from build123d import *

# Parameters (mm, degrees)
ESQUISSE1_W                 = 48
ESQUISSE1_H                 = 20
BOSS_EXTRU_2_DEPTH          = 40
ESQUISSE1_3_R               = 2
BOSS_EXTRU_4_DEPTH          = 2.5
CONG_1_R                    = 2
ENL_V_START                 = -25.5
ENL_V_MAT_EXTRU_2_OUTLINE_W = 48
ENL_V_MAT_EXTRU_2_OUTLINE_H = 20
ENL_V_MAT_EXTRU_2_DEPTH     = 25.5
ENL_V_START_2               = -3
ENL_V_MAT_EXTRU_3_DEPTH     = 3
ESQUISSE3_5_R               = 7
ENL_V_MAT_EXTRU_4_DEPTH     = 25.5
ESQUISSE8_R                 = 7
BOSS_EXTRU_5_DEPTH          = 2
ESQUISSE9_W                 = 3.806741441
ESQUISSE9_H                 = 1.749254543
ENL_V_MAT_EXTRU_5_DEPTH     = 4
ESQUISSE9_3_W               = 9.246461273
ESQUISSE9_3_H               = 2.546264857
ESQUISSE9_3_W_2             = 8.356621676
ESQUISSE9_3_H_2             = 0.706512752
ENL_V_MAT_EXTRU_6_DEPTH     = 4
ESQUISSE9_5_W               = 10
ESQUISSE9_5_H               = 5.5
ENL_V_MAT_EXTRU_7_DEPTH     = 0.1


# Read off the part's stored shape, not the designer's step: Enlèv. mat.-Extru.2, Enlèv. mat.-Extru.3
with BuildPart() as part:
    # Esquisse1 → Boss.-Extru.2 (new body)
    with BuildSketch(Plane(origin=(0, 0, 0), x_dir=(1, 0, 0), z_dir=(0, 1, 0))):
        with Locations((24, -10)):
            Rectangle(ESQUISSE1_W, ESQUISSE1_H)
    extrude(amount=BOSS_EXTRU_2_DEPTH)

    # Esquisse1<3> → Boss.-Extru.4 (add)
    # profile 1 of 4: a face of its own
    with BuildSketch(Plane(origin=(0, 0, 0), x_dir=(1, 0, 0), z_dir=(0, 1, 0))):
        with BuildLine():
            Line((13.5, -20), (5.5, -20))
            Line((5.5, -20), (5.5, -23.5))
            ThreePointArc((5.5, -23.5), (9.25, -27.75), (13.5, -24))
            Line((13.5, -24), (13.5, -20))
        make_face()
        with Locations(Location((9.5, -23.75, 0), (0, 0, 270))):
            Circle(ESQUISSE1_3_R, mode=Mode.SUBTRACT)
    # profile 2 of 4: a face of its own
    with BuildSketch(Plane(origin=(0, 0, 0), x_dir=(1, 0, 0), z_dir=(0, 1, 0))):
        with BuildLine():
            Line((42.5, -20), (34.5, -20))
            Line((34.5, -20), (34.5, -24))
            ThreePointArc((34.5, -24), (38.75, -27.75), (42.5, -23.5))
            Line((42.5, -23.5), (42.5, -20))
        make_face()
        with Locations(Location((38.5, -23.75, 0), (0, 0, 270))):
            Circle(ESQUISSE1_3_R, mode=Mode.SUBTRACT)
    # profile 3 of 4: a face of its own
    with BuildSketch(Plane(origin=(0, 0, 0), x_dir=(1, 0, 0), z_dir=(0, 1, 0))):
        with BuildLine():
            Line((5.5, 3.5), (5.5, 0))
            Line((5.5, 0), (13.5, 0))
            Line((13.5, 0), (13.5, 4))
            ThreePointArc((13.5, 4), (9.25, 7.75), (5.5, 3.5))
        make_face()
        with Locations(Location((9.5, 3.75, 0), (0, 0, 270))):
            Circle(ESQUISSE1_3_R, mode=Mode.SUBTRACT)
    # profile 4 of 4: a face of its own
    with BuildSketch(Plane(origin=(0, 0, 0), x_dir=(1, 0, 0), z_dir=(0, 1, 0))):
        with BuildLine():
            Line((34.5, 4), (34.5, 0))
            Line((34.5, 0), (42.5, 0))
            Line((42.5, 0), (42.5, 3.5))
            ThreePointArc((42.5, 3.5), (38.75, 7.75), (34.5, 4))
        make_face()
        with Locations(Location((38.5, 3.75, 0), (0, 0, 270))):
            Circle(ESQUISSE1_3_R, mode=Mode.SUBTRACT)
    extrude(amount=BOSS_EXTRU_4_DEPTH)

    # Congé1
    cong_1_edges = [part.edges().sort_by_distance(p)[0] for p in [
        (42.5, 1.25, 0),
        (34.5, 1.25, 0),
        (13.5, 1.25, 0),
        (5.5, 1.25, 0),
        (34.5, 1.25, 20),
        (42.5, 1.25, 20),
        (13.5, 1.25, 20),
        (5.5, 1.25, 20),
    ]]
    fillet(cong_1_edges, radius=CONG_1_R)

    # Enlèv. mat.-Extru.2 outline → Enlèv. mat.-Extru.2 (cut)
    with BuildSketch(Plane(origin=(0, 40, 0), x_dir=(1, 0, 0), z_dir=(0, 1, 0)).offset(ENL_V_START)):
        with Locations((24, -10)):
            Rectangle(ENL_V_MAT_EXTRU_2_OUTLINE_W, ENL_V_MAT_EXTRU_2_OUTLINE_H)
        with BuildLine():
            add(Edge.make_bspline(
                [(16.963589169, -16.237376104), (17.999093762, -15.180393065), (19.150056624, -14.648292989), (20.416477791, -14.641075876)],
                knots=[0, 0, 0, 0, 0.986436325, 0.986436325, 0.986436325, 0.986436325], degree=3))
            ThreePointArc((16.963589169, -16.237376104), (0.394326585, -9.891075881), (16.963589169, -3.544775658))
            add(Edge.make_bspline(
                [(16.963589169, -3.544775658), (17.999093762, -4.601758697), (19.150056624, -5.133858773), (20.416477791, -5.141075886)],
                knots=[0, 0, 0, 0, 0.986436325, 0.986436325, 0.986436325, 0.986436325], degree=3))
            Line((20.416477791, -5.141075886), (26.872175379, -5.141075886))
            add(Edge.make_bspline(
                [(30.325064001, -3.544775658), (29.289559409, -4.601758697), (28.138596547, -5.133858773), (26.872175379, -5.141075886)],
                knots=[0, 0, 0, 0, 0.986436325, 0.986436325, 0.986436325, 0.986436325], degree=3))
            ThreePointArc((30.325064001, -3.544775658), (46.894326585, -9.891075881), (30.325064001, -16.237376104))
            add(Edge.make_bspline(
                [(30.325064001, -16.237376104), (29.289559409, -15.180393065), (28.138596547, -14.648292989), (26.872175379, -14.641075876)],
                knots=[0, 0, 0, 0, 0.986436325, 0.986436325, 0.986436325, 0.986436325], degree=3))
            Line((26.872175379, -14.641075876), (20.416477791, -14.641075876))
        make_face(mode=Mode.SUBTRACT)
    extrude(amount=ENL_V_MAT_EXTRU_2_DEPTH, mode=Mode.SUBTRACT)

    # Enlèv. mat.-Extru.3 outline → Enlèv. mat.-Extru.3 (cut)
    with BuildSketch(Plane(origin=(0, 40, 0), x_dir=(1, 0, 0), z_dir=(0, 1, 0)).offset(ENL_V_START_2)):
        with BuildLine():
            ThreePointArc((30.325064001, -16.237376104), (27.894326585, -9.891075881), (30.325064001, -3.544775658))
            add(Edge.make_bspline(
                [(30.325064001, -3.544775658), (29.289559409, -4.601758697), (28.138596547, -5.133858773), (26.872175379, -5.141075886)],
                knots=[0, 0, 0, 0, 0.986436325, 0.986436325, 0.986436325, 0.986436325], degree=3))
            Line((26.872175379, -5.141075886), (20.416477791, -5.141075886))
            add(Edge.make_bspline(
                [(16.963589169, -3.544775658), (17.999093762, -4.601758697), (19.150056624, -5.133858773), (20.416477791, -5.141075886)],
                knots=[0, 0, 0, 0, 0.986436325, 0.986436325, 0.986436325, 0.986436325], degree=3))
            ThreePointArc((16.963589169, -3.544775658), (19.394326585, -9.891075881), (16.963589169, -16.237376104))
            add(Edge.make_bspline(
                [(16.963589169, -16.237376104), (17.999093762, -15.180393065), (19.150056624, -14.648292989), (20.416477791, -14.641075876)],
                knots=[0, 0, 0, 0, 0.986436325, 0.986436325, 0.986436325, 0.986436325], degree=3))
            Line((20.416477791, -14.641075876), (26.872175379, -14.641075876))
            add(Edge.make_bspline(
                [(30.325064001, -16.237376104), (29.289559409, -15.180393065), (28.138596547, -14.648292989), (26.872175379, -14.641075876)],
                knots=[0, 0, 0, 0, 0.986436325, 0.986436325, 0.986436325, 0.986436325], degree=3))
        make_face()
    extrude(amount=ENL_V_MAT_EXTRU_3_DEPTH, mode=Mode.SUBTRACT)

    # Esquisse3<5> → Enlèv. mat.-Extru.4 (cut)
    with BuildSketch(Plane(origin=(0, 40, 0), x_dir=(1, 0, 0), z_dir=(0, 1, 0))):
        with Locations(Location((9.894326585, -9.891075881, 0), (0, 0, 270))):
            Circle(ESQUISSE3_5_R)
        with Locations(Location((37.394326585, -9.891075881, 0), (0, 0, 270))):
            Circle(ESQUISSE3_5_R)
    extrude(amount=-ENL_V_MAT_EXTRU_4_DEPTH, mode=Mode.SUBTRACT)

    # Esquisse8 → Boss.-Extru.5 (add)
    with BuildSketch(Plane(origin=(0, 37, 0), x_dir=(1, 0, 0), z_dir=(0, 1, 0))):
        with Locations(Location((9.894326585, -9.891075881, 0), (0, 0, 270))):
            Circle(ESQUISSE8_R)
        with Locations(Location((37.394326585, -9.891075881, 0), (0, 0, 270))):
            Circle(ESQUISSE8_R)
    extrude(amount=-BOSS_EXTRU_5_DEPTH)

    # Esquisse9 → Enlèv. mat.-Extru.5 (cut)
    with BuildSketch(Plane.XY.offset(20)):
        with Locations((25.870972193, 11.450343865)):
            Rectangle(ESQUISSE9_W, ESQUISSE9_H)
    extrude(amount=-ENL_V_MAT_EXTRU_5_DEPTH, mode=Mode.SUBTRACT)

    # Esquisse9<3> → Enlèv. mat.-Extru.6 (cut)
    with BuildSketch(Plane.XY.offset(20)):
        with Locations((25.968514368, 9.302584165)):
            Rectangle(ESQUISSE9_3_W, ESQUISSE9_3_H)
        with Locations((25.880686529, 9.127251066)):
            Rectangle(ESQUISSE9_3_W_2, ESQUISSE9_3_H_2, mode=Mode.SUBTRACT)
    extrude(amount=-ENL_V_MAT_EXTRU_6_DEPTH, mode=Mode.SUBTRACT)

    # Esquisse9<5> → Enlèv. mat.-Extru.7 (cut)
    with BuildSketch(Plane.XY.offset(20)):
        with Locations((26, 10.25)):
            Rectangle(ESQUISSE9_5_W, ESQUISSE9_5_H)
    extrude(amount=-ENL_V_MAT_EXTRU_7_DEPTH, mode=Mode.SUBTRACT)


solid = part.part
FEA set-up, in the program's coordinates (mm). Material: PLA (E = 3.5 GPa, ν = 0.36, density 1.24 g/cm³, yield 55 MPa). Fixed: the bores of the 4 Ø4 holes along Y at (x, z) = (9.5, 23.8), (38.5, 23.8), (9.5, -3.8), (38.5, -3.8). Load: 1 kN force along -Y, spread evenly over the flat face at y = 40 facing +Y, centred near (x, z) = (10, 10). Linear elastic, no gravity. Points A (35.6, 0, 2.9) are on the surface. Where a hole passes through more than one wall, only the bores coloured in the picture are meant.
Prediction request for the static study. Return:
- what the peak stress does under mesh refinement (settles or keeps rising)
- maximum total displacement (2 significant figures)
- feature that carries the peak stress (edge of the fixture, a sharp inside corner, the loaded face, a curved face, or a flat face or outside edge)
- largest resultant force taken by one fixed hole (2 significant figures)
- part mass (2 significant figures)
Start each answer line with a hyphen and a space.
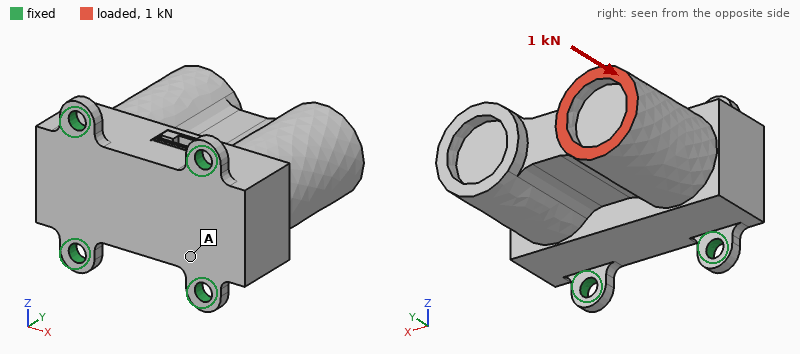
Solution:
- keeps rising
- 0.32 mm
- edge of the fixture
- 540 N
- 29 g
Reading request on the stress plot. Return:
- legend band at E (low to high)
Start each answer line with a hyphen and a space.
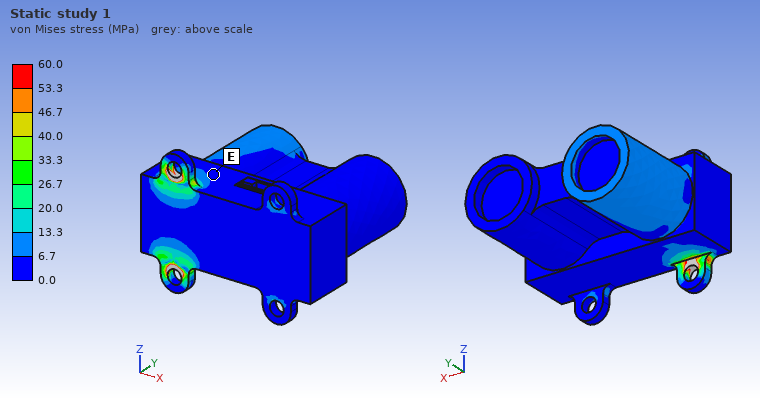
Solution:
- 0.0 to 6.7 MPa
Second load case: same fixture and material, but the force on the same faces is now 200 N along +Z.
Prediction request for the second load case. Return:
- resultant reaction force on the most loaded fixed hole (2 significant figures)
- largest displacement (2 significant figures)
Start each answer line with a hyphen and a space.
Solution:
- 220 N
- 0.32 mm
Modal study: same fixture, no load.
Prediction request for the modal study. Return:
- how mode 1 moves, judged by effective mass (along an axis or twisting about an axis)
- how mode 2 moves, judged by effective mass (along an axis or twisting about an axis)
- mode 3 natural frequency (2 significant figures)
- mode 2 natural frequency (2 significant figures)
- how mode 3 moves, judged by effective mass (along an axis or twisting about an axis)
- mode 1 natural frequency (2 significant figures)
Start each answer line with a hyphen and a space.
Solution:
- along Z
- along X
- 3500 Hz
- 2100 Hz
- along Y
- 1900 Hz
